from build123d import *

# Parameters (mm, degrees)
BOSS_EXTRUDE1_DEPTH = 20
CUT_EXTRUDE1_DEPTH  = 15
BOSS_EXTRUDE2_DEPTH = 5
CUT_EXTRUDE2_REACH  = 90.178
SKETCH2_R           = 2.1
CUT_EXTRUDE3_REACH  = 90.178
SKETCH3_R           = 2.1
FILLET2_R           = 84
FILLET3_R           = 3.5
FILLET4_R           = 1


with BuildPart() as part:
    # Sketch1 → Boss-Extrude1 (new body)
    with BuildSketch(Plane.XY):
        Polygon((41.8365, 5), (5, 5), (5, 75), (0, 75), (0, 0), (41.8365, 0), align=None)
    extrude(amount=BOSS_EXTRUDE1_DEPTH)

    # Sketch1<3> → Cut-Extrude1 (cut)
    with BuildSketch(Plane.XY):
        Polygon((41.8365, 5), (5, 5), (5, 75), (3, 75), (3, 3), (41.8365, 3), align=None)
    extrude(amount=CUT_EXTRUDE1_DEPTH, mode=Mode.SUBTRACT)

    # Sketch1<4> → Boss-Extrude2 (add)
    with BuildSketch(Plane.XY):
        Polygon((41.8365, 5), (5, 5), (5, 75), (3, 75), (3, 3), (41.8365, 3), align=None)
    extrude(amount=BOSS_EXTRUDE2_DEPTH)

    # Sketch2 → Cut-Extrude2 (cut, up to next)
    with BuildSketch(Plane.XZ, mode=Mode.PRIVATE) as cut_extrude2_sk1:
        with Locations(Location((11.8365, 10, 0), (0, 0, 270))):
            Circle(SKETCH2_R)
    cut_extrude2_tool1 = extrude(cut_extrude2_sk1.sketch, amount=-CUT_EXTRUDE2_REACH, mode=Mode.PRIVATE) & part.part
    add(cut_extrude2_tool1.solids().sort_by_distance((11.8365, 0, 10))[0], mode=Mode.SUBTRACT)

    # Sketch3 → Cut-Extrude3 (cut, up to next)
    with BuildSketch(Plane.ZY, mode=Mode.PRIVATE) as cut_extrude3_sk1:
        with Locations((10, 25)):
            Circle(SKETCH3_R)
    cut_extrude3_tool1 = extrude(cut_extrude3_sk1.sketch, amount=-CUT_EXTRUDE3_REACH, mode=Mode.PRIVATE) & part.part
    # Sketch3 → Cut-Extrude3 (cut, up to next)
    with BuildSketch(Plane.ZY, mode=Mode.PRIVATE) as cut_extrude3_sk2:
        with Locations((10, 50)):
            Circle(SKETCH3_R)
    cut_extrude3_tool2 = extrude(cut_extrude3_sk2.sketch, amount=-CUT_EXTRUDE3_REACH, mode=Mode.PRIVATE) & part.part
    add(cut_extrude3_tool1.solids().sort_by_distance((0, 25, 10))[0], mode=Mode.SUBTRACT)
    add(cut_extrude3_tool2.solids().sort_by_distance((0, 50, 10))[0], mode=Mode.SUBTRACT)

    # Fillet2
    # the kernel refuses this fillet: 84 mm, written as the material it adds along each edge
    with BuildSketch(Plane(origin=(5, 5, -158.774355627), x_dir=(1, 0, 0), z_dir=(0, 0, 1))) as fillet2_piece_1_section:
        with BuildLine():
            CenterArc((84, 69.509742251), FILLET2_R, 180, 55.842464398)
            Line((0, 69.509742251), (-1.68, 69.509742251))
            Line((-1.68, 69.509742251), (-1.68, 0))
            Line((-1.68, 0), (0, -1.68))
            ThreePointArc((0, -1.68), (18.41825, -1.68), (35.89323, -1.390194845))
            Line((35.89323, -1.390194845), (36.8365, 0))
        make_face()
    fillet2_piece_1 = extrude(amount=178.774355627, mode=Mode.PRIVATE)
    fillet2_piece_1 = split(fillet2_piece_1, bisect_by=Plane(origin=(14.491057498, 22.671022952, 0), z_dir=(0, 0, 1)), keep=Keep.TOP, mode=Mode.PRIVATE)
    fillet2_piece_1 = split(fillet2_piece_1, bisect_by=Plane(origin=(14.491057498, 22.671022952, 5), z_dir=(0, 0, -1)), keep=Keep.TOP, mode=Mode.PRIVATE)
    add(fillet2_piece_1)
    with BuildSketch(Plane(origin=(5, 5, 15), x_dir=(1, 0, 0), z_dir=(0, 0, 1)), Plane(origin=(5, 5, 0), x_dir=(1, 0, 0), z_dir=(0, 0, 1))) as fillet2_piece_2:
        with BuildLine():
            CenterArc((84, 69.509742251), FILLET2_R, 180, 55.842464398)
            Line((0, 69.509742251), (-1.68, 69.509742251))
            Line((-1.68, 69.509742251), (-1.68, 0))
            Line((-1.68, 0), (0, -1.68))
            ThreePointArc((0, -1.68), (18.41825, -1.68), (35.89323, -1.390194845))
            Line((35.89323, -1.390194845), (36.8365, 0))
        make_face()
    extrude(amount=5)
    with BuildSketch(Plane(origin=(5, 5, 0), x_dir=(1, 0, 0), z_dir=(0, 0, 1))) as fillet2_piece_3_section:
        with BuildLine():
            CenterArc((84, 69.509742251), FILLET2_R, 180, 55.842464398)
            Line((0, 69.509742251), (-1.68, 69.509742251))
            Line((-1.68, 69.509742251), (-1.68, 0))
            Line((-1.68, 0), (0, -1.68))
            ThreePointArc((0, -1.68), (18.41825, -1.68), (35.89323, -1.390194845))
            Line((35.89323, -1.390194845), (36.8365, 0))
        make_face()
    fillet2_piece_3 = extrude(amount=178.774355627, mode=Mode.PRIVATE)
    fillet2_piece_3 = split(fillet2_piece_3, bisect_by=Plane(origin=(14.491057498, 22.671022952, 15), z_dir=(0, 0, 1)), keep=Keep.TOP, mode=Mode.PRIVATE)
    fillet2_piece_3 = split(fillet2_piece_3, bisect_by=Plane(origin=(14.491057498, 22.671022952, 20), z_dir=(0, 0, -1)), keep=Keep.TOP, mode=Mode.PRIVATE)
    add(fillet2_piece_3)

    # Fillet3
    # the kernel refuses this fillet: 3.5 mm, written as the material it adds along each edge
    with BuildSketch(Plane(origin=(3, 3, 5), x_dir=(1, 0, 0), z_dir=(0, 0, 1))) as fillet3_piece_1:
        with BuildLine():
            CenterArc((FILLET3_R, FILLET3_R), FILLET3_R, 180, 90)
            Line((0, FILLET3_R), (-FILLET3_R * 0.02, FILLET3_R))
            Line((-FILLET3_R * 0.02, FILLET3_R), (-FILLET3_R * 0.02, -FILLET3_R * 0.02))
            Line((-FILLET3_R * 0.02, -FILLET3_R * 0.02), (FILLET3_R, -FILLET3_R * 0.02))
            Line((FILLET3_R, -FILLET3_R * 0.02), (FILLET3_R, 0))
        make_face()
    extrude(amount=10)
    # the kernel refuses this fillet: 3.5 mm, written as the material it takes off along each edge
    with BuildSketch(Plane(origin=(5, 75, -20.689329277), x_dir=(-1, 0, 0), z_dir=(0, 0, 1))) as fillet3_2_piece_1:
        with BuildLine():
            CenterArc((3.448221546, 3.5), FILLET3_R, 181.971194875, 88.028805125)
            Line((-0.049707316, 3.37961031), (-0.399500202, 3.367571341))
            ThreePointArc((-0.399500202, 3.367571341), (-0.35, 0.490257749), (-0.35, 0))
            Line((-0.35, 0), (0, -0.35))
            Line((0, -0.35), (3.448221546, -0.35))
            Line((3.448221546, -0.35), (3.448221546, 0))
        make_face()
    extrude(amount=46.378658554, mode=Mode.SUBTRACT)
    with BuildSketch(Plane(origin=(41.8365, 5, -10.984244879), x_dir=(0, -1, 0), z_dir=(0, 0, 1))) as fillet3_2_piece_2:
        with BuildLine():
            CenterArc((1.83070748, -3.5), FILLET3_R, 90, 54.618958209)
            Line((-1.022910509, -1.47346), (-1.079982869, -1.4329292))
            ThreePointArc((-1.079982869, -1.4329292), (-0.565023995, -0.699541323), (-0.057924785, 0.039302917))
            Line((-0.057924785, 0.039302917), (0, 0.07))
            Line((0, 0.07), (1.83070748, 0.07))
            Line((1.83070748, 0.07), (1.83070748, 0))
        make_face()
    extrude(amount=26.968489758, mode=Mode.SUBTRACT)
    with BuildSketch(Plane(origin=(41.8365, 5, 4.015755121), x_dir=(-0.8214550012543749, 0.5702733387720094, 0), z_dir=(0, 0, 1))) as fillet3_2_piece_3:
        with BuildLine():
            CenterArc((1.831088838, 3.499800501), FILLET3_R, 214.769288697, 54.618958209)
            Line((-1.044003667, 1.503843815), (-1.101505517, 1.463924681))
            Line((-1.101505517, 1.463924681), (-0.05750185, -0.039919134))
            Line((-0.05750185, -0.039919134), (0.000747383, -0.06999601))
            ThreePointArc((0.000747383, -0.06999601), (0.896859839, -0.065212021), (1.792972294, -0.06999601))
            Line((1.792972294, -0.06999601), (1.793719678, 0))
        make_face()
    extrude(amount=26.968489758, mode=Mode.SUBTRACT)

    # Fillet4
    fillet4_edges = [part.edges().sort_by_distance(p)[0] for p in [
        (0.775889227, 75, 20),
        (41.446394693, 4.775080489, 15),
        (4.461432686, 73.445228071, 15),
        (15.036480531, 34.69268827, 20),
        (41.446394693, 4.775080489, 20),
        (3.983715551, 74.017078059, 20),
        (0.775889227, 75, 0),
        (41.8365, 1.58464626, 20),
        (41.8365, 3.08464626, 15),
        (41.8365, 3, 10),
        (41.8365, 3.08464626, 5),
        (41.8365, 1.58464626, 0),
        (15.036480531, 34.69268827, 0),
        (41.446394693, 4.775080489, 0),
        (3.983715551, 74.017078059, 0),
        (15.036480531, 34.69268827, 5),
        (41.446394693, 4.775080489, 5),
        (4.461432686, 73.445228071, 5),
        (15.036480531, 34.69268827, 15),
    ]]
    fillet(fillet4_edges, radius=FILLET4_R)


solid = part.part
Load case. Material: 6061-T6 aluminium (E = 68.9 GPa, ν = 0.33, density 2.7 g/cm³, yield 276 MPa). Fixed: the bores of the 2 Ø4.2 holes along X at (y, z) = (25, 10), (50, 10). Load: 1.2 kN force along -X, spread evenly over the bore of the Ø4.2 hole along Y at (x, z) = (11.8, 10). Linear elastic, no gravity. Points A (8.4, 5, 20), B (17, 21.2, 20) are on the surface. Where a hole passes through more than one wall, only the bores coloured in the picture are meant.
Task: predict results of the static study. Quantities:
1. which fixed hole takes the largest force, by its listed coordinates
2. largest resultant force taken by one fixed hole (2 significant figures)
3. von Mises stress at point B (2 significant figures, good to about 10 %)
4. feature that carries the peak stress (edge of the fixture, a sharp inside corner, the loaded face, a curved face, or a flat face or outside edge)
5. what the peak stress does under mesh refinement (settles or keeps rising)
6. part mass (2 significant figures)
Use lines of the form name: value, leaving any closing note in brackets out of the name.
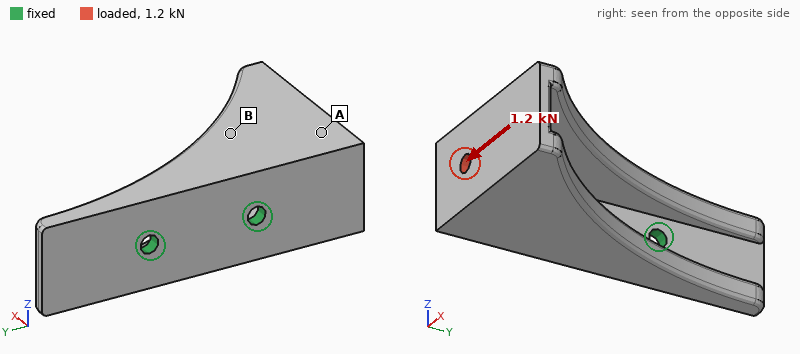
which fixed hole takes the largest force, by its listed coordinates: (25, 10)
largest resultant force taken by one fixed hole: 2.3 kN
von Mises stress at point B: 22 MPa
feature that carries the peak stress: edge of the fixture
what the peak stress does under mesh refinement: keeps rising
part mass: 44 g
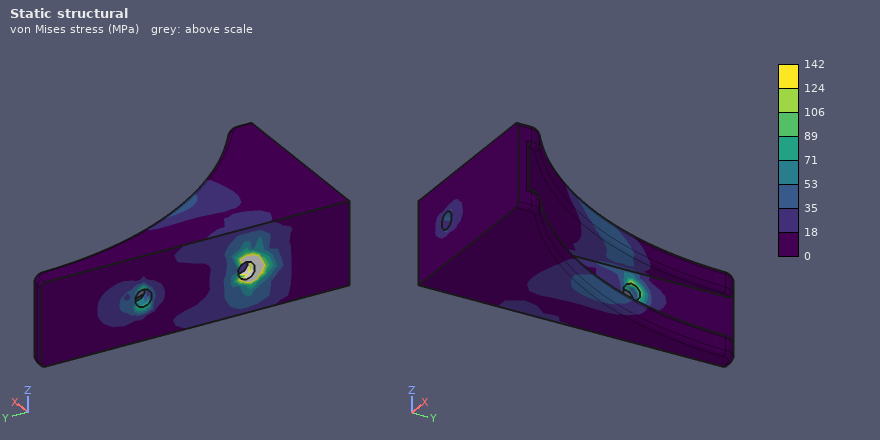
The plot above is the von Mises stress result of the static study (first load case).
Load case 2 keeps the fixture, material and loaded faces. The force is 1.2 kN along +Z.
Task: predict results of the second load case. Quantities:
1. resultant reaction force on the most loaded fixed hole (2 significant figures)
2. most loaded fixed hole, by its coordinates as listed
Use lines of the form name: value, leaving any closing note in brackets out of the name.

resultant reaction force on the most loaded fixed hole: 2.1 kN
most loaded fixed hole, by its coordinates as listed: (25, 10)
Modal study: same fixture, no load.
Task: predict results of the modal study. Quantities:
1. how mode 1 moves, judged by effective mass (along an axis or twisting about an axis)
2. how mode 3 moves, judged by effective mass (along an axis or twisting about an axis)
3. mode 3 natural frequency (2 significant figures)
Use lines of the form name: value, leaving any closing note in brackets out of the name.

how mode 1 moves, judged by effective mass: along Z
how mode 3 moves, judged by effective mass: along X
mode 3 natural frequency: 8000 Hz
